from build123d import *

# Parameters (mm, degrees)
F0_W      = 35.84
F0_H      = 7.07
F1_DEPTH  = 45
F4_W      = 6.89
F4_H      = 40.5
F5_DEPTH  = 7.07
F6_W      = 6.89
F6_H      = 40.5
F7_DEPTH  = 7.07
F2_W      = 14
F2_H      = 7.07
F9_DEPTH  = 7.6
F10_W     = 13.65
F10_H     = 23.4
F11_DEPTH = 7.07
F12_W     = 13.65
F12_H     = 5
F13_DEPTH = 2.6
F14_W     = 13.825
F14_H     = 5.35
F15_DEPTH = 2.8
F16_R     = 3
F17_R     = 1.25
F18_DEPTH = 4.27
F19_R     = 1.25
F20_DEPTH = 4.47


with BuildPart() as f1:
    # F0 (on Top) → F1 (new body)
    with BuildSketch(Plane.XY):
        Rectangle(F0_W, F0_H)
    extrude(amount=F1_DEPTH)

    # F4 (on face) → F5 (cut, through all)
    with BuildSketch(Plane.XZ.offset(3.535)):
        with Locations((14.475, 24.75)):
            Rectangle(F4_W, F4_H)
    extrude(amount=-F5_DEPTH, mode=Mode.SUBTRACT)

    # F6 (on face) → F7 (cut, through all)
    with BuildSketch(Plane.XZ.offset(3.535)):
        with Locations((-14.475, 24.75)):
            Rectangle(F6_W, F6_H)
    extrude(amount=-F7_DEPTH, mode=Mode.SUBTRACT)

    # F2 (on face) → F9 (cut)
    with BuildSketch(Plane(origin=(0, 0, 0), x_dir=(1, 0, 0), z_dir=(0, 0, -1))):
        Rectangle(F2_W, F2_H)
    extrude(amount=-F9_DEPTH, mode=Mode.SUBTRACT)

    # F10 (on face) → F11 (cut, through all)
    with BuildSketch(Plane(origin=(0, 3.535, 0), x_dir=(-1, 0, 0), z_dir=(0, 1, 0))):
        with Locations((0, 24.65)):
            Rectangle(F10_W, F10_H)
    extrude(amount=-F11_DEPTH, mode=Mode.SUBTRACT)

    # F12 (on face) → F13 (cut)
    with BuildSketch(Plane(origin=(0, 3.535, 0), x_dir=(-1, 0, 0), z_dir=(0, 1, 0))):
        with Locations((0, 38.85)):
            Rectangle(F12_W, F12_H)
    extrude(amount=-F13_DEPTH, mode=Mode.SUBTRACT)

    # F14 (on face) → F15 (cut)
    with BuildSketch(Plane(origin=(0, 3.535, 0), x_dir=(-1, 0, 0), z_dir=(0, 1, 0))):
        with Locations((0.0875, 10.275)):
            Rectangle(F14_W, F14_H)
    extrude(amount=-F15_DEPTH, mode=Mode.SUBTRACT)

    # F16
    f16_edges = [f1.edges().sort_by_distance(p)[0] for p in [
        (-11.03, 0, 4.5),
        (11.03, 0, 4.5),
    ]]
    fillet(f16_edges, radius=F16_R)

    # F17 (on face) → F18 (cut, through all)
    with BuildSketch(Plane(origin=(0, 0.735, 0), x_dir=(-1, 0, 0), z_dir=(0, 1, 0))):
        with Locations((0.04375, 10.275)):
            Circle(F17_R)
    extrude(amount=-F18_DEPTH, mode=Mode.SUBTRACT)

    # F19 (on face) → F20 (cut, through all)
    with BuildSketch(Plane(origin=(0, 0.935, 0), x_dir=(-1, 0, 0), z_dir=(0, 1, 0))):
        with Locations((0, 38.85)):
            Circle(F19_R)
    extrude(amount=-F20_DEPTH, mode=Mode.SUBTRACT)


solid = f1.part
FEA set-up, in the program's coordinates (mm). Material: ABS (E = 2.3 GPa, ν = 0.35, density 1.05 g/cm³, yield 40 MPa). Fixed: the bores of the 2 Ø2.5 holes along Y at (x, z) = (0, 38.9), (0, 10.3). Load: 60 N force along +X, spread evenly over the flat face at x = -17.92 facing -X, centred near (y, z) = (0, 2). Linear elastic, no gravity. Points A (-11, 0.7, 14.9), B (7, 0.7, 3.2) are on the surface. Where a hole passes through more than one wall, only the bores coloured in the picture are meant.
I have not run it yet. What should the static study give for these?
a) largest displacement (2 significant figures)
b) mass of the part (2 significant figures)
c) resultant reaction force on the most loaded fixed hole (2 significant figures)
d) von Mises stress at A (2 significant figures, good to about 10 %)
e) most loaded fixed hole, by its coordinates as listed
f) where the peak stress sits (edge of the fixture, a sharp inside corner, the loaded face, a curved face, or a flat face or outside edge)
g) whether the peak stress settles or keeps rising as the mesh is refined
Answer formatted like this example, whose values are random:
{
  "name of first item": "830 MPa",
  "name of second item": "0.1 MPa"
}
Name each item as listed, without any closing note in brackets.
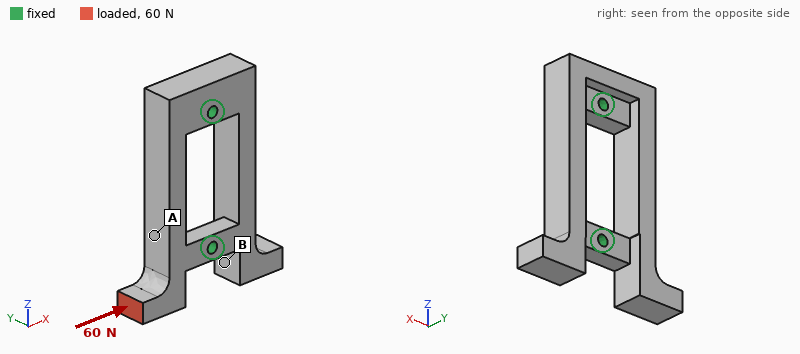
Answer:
{
  "largest displacement": "0.41 mm",
  "mass of the part": "4.2 g",
  "resultant reaction force on the most loaded fixed hole": "78 N",
  "von Mises stress at A": "6.7 MPa",
  "most loaded fixed hole, by its coordinates as listed": "(0, 10.3)",
  "where the peak stress sits": "a sharp inside corner",
  "whether the peak stress settles or keeps rising as the mesh is refined": "keeps rising"
}
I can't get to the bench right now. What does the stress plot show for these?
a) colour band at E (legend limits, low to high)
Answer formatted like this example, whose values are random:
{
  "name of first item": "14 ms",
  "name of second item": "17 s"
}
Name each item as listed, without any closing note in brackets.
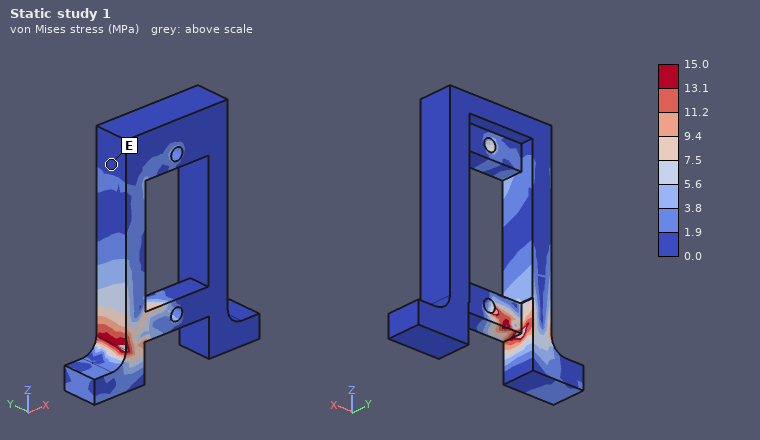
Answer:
{
  "colour band at E": "0.0 to 1.9 MPa"
}
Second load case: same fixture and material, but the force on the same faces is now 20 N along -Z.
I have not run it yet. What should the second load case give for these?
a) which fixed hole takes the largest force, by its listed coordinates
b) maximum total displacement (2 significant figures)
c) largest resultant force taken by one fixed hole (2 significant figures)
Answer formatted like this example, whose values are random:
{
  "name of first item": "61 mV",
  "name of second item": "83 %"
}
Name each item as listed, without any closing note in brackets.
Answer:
{
  "which fixed hole takes the largest force, by its listed coordinates": "(0, 38.9)",
  "maximum total displacement": "0.23 mm",
  "largest resultant force taken by one fixed hole": "25 N"
}
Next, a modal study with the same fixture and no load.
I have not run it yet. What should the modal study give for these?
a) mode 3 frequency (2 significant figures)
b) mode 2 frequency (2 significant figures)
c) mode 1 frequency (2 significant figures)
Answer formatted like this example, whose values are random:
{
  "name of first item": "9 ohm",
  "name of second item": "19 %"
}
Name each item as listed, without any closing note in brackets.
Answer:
{
  "mode 3 frequency": "3000 Hz",
  "mode 2 frequency": "2200 Hz",
  "mode 1 frequency": "2200 Hz"
}
